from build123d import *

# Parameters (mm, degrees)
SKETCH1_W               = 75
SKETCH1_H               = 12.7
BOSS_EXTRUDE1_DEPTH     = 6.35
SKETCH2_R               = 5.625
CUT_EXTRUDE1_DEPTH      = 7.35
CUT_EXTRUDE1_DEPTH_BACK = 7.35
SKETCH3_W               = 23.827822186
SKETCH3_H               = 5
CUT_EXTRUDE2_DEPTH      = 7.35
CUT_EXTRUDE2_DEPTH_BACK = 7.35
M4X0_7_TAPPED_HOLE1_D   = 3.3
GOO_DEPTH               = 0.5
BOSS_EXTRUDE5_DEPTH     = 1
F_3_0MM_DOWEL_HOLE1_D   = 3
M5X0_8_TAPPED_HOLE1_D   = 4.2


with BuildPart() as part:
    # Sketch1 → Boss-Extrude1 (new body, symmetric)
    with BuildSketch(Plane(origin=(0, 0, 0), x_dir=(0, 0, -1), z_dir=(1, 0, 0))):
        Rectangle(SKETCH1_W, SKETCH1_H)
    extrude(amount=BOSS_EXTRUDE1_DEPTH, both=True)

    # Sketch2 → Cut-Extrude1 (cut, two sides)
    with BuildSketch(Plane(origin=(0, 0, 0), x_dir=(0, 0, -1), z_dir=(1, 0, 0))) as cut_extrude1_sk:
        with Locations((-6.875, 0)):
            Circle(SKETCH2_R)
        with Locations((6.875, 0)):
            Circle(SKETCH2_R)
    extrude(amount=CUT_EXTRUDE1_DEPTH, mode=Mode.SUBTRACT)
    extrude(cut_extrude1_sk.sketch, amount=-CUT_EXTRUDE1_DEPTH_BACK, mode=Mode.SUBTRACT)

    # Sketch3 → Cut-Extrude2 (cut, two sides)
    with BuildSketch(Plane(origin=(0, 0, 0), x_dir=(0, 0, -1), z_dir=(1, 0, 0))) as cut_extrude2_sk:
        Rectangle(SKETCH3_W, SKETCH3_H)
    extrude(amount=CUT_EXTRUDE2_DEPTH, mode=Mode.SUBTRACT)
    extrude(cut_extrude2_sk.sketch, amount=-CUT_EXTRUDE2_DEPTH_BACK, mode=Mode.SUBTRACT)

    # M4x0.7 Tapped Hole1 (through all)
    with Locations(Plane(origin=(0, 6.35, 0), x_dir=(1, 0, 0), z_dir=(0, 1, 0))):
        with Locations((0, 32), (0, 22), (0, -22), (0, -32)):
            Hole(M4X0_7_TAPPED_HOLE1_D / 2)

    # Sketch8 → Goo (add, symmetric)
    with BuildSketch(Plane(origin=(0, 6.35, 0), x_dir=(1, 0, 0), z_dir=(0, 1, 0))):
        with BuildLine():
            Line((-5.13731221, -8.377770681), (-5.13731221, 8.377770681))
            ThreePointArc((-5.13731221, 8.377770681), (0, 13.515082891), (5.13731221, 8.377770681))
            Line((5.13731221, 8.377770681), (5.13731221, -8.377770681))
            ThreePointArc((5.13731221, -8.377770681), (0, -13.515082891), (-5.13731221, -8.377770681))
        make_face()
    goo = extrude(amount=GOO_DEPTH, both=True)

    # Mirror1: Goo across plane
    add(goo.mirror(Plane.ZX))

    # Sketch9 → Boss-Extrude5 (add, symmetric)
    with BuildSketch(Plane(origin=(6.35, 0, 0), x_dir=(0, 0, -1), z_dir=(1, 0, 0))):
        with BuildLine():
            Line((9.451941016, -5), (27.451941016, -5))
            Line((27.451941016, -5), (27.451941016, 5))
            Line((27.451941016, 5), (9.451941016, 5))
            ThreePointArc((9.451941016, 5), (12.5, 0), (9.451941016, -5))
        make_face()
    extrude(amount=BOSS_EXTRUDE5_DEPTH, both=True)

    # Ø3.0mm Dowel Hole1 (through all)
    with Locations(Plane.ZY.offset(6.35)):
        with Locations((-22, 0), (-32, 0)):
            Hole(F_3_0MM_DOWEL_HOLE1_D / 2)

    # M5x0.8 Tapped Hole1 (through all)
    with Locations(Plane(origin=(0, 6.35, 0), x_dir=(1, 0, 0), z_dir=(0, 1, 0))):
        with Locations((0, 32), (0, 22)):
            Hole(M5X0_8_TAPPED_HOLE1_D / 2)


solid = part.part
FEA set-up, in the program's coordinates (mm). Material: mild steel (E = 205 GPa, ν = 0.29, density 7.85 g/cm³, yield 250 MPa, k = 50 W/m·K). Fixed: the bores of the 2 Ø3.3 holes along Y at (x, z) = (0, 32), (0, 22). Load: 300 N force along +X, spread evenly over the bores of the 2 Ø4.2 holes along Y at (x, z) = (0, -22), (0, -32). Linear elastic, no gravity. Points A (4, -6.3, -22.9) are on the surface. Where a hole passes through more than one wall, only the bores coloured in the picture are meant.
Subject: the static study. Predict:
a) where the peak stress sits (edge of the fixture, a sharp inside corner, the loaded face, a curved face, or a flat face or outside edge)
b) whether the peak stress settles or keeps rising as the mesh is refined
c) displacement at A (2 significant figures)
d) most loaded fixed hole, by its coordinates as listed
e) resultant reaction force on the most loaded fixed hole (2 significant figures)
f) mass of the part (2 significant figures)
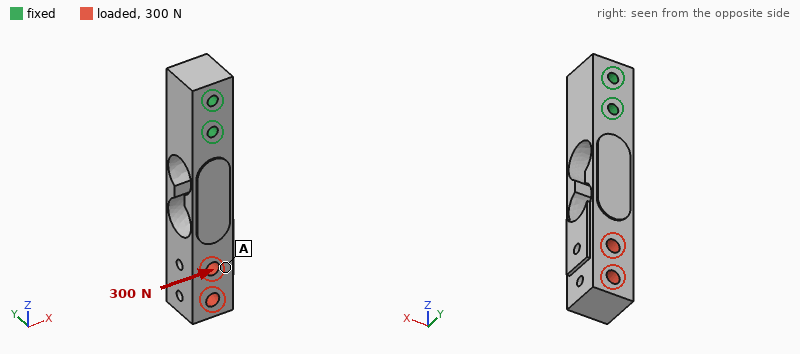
a sharp inside corner
keeps rising
0.084 mm
(0, 22)
1.1 kN
71 g
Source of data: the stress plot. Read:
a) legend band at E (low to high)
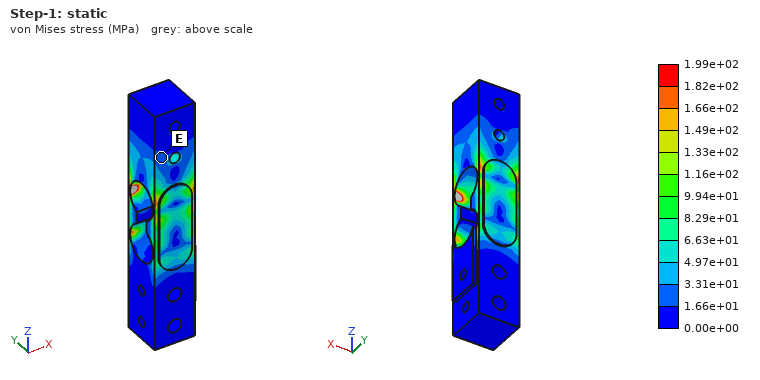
1.66e+01 to 3.31e+01 MPa
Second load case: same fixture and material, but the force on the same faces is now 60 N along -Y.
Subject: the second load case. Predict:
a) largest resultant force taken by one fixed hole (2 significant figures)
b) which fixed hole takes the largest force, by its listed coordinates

100 N
(0, 22)
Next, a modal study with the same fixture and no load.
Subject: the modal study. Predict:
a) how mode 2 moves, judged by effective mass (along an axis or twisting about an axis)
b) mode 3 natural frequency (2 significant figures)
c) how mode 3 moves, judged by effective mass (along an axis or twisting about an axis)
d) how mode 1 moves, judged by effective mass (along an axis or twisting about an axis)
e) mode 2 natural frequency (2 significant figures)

along X
5800 Hz
twisting about Z
along Y
1700 Hz
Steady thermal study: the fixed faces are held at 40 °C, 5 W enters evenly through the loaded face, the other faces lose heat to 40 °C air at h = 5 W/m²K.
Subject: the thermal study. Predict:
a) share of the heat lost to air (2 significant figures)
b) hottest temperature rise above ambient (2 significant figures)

15 %
64 K
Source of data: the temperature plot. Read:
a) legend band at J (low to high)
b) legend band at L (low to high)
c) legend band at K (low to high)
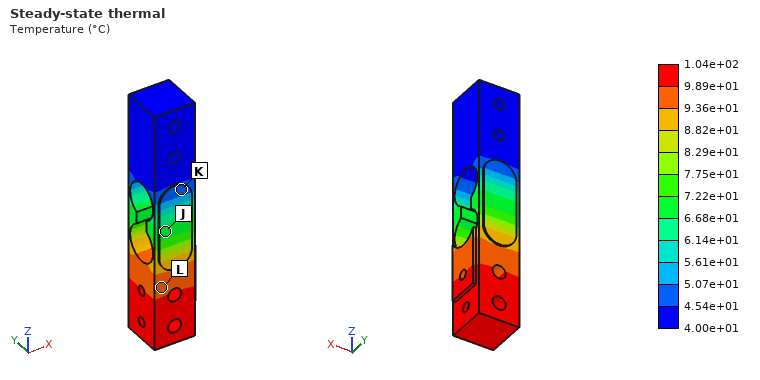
6.68e+01 to 7.22e+01 °C
9.36e+01 to 9.89e+01 °C
4.54e+01 to 5.07e+01 °C
